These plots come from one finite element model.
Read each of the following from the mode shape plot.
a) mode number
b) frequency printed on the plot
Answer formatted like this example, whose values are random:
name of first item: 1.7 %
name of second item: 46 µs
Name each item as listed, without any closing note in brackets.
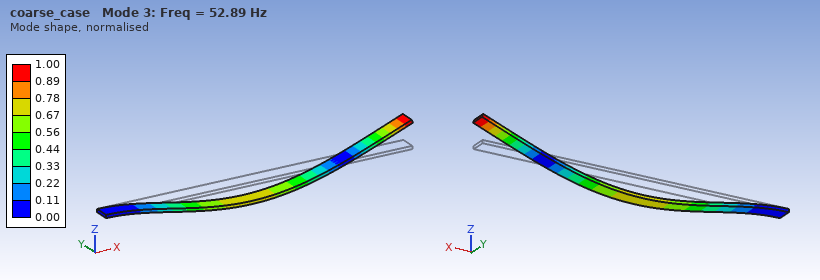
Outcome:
mode number: 3
frequency printed on the plot: 52.89 Hz
